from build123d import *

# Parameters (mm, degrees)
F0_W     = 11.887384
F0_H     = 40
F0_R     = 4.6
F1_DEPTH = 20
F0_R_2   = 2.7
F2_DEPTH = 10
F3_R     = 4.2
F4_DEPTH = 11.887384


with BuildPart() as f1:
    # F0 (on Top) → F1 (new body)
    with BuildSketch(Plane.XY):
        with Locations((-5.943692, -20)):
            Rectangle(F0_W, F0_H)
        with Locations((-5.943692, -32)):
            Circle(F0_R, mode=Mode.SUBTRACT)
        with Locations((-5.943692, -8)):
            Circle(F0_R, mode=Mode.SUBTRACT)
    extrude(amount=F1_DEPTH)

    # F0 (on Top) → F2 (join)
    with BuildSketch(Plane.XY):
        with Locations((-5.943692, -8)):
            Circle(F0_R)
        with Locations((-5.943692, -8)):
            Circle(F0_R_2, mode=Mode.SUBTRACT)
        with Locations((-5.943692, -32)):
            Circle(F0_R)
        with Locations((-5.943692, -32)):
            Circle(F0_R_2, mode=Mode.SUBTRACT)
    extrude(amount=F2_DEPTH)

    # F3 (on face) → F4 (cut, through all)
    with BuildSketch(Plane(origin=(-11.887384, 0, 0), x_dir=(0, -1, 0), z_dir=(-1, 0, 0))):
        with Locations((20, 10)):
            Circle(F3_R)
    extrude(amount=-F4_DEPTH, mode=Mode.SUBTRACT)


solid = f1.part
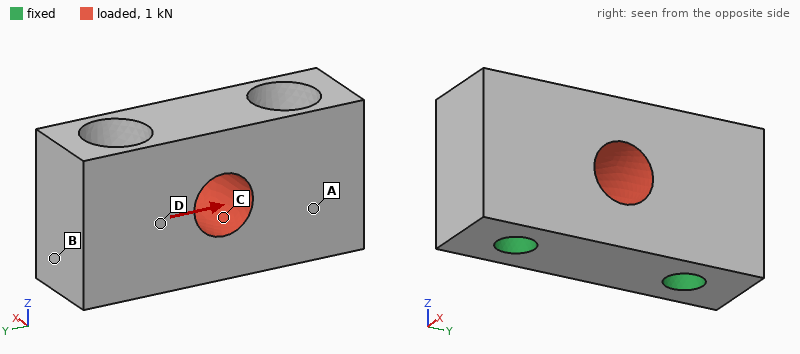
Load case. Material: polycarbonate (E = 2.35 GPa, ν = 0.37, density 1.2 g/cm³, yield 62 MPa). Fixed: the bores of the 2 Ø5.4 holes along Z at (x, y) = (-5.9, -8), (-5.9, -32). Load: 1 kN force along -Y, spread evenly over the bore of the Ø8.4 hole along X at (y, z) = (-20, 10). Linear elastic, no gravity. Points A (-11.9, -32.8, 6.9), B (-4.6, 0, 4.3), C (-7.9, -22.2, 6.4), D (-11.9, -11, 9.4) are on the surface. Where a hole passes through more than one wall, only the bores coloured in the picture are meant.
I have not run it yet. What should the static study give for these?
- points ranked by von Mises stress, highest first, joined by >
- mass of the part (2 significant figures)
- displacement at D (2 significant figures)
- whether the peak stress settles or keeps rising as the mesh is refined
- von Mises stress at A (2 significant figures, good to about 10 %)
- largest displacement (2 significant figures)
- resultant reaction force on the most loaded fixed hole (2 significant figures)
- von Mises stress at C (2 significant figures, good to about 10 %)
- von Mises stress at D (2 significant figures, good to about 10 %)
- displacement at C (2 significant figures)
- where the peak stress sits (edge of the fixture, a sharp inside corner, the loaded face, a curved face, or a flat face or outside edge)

C > D > A > B
8.5 g
14 µm
keeps rising
2.4 MPa
42 µm
510 N
5.6 MPa
3.9 MPa
13 µm
a sharp inside corner
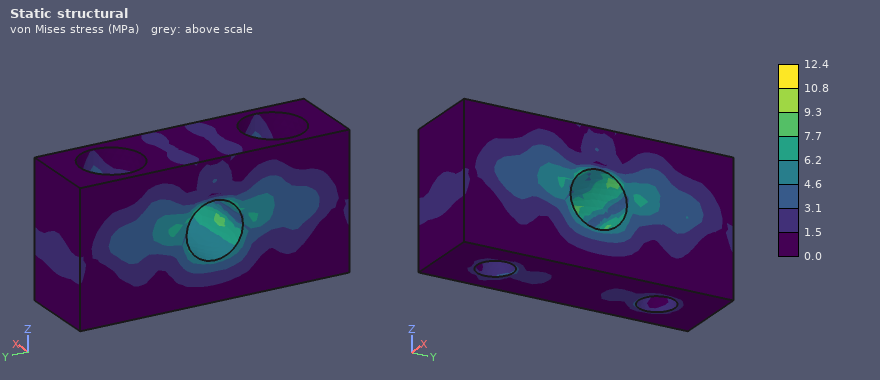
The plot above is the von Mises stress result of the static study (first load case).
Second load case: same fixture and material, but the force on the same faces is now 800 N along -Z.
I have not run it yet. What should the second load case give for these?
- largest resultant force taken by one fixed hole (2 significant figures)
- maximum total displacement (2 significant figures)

410 N
36 µm
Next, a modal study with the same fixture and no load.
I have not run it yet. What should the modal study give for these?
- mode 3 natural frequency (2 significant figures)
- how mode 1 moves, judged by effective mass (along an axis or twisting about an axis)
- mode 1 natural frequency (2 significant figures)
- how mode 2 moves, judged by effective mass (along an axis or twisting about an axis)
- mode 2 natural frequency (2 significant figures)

9800 Hz
along X
6800 Hz
twisting about Z
9200 Hz
